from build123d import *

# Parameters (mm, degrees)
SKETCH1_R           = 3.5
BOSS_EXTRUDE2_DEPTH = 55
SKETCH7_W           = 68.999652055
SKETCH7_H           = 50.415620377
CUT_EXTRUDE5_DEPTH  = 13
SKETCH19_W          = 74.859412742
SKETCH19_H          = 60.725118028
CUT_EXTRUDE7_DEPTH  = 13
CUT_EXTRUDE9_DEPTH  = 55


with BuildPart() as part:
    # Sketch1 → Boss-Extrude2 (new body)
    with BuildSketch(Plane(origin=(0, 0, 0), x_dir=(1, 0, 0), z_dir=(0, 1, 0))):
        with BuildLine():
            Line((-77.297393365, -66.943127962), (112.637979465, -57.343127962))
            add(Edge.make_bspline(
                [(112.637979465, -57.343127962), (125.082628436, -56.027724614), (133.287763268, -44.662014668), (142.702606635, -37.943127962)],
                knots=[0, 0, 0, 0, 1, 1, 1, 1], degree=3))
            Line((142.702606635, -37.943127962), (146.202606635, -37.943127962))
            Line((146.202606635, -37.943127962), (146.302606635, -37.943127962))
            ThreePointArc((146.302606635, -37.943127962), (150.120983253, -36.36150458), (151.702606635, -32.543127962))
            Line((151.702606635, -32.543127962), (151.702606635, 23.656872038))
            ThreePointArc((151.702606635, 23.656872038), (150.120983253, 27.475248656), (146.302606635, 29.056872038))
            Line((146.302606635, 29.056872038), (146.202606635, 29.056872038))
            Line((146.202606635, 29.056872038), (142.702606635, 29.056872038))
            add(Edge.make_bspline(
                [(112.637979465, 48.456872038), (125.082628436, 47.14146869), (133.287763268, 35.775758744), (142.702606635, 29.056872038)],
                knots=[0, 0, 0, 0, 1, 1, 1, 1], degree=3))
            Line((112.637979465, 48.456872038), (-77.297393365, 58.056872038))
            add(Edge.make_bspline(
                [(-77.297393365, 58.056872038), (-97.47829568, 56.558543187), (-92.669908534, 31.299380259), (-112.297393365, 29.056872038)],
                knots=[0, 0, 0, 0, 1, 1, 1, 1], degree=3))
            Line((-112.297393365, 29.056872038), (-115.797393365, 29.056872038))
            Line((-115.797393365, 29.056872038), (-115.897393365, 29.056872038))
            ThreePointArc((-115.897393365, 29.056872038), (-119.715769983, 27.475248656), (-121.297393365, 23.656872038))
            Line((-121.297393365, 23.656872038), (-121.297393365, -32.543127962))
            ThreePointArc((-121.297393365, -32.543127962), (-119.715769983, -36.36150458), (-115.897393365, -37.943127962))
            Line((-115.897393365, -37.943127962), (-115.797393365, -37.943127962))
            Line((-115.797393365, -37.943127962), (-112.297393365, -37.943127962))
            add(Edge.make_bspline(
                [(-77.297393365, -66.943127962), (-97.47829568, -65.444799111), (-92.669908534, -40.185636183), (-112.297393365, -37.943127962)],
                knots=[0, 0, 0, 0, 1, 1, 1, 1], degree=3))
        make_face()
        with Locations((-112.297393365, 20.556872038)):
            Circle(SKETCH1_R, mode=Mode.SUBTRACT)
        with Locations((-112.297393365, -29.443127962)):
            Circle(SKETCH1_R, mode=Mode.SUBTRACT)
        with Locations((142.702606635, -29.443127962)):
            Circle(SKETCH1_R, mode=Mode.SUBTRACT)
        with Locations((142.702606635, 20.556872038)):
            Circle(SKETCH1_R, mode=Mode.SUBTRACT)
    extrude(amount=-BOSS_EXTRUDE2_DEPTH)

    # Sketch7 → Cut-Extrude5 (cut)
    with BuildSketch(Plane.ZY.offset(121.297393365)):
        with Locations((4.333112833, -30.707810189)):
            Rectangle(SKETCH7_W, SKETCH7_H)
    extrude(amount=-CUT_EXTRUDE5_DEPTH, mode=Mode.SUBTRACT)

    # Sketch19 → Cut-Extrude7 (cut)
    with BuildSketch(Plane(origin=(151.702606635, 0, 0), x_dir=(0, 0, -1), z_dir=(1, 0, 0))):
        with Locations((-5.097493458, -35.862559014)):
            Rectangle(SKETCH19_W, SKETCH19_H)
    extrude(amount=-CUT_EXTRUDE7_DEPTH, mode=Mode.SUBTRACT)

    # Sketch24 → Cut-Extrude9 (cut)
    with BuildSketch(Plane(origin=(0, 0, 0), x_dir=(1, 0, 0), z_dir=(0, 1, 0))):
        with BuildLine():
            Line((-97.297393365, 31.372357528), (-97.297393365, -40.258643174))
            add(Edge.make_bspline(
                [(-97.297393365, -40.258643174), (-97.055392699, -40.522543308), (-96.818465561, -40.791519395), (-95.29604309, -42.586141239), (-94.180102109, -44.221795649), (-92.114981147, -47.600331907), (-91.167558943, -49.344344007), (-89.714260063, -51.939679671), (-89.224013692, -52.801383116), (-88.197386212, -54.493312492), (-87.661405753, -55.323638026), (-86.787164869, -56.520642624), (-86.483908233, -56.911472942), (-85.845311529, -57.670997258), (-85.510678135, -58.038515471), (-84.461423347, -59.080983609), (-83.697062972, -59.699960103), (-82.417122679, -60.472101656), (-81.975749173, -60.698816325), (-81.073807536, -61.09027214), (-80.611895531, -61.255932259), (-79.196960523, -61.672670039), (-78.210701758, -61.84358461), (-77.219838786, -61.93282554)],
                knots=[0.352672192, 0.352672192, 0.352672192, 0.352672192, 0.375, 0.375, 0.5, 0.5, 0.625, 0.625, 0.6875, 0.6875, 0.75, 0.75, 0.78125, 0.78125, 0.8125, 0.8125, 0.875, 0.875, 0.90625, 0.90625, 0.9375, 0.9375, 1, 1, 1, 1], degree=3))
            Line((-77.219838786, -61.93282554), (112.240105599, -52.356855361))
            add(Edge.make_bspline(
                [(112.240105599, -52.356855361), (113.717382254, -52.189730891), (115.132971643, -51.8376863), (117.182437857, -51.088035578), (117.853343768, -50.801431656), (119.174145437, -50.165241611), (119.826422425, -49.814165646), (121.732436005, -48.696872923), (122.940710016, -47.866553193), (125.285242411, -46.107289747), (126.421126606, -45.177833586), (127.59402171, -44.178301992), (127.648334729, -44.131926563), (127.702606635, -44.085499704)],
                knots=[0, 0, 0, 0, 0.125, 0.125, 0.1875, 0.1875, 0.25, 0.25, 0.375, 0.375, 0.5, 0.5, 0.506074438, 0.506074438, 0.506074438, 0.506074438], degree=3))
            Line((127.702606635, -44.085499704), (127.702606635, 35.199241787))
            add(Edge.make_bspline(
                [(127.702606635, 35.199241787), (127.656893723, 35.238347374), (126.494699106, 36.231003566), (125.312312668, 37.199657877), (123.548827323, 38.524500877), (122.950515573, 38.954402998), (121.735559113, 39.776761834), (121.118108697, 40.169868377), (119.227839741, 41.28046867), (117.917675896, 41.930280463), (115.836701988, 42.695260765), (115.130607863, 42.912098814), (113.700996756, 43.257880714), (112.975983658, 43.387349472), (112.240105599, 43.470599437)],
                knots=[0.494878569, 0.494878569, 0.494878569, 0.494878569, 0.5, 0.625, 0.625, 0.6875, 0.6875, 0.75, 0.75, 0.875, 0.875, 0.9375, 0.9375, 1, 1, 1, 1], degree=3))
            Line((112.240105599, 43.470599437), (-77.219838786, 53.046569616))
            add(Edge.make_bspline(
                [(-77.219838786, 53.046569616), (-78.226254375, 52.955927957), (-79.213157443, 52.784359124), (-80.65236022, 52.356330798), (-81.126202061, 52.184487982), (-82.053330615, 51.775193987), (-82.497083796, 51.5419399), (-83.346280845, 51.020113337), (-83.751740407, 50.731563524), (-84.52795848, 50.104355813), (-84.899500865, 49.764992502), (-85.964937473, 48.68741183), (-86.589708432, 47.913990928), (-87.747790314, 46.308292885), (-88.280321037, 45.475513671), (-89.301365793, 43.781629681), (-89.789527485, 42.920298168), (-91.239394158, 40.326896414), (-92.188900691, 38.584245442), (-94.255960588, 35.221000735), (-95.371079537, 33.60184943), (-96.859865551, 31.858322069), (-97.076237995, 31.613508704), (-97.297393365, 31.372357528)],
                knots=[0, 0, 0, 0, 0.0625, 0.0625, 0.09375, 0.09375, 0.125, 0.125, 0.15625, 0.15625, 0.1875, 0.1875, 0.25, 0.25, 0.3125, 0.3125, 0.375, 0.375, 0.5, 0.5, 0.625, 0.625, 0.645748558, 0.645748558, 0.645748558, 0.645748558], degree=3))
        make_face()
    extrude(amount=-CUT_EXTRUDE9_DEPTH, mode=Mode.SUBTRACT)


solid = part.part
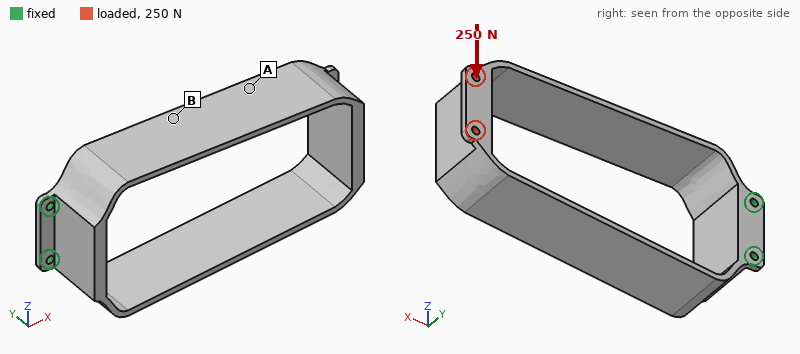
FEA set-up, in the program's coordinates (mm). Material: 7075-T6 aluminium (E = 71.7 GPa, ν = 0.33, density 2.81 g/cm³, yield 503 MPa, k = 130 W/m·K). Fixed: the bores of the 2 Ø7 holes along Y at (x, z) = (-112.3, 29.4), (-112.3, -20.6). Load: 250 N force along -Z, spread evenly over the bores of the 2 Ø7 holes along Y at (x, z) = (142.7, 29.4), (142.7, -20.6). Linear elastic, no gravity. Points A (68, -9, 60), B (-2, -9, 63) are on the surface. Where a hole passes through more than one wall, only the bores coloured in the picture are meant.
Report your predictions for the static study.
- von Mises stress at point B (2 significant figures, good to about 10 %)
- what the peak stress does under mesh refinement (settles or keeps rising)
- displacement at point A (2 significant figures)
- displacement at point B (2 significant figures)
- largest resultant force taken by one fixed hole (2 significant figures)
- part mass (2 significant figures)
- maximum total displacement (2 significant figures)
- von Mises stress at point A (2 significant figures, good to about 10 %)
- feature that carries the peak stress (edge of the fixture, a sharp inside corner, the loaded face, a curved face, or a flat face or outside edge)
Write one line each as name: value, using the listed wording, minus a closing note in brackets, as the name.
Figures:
von Mises stress at point B: 10 MPa
what the peak stress does under mesh refinement: keeps rising
displacement at point A: 3.0 mm
displacement at point B: 1.6 mm
largest resultant force taken by one fixed hole: 1.1 kN
part mass: 660 g
maximum total displacement: 3.6 mm
von Mises stress at point A: 28 MPa
feature that carries the peak stress: edge of the fixture
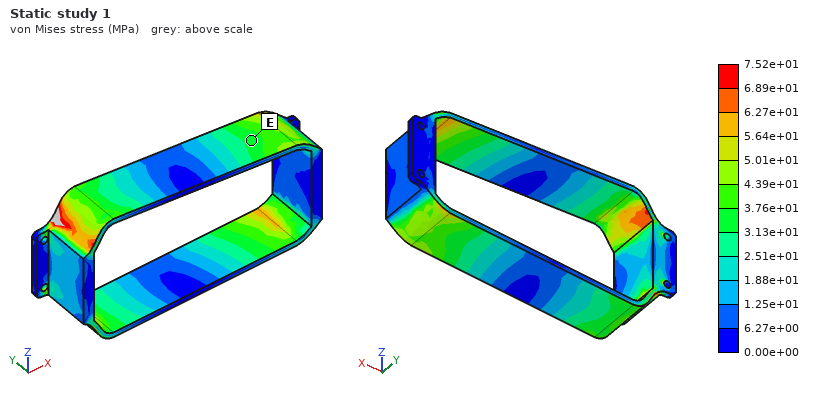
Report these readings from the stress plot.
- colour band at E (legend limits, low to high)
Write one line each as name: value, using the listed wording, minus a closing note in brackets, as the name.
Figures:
colour band at E: 3.13e+01 to 3.76e+01 MPa
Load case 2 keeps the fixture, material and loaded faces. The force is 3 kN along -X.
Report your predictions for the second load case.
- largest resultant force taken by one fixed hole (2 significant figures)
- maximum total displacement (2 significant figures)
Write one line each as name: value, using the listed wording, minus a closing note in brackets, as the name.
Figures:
largest resultant force taken by one fixed hole: 2.4 kN
maximum total displacement: 2.0 mm
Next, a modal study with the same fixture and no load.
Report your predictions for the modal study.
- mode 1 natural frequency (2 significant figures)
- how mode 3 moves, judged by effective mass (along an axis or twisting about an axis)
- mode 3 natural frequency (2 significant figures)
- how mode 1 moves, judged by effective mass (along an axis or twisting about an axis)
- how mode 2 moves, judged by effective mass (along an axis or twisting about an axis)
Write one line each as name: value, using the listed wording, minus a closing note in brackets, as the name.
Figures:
mode 1 natural frequency: 79 Hz
how mode 3 moves, judged by effective mass: twisting about X
mode 3 natural frequency: 380 Hz
how mode 1 moves, judged by effective mass: along Z
how mode 2 moves, judged by effective mass: along Y
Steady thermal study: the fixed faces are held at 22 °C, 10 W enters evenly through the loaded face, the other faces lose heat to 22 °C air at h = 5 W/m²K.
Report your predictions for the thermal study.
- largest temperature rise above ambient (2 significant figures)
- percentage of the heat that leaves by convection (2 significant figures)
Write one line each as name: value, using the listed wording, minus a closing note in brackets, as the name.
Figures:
largest temperature rise above ambient: 28 K
percentage of the heat that leaves by convection: 50 %
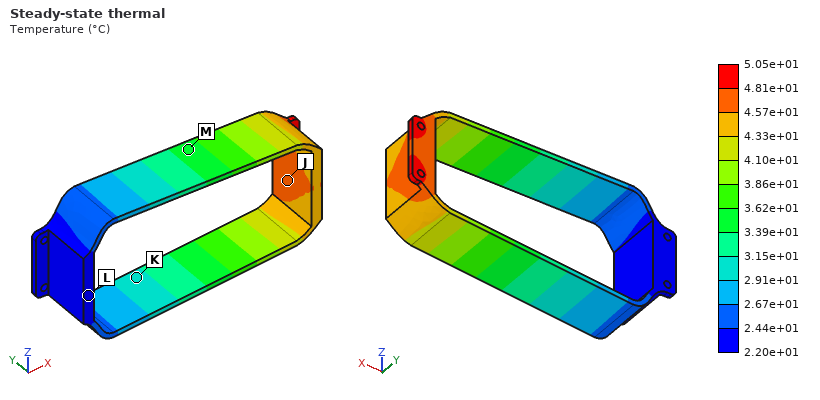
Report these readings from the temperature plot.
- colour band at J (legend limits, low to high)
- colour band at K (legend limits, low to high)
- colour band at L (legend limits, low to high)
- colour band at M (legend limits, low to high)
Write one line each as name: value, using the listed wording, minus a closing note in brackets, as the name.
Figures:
colour band at J: 4.57e+01 to 4.81e+01 °C
colour band at K: 2.91e+01 to 3.15e+01 °C
colour band at L: 2.20e+01 to 2.44e+01 °C
colour band at M: 3.39e+01 to 3.62e+01 °C
